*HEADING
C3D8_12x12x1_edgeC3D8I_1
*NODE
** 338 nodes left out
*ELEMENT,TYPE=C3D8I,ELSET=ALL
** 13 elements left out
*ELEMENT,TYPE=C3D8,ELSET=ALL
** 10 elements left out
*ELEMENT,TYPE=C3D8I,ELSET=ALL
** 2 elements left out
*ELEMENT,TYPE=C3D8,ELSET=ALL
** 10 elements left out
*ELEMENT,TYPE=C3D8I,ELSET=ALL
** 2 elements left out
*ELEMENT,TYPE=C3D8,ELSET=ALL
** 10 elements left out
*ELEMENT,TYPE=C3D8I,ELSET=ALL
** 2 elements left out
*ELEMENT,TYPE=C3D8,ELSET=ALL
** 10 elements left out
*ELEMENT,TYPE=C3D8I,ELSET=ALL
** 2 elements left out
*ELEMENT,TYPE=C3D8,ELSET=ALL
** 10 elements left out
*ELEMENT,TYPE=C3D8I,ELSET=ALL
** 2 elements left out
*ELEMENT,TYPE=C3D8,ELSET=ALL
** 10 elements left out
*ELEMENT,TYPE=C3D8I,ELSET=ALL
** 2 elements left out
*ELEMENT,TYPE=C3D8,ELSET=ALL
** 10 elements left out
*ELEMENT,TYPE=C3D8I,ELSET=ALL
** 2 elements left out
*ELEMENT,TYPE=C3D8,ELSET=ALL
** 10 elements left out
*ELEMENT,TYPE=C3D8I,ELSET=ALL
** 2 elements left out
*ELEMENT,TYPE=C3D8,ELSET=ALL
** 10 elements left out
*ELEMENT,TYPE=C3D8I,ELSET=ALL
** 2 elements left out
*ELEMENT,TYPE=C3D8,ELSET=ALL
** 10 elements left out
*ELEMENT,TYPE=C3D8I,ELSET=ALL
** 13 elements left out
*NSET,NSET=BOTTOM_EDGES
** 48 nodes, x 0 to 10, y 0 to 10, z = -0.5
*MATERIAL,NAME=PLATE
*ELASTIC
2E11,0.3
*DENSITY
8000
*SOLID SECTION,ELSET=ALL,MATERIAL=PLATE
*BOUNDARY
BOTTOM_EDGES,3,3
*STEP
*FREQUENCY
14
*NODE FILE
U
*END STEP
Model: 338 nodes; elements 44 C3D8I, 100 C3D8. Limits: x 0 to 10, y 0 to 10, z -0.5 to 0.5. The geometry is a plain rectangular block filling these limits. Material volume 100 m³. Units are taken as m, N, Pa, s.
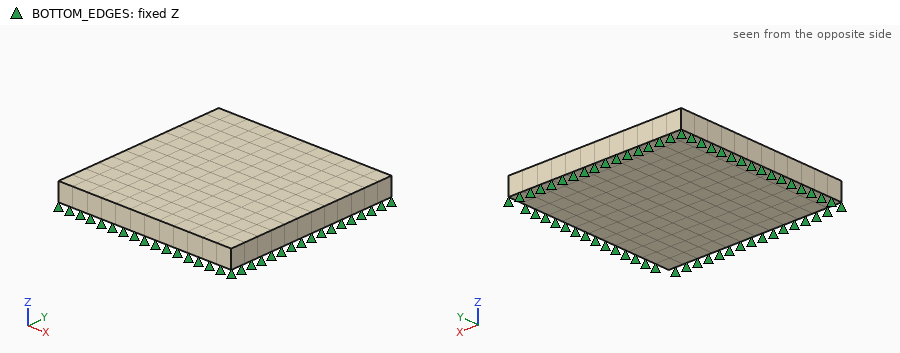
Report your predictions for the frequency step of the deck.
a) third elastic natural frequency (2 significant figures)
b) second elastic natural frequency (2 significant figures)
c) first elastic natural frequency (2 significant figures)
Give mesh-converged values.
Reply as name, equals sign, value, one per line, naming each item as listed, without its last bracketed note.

third elastic natural frequency = 100 Hz
second elastic natural frequency = 100 Hz
first elastic natural frequency = 43 Hz
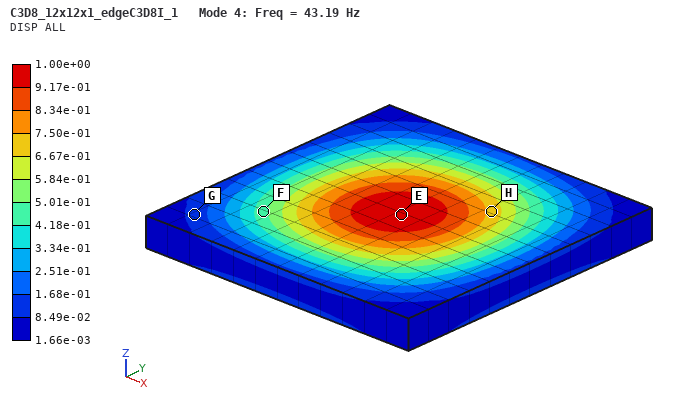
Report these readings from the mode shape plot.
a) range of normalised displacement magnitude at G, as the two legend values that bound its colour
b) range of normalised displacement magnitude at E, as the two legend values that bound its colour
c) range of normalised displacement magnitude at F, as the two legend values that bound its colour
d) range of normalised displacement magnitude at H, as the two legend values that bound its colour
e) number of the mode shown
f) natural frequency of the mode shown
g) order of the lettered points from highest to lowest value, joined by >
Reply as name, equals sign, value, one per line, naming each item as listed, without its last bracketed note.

range of normalised displacement magnitude at G, as the two legend values that bound its colour = 8.49e-02 to 1.68e-01
range of normalised displacement magnitude at E, as the two legend values that bound its colour = 9.17e-01 to 1.00e+00
range of normalised displacement magnitude at F, as the two legend values that bound its colour = 4.18e-01 to 5.01e-01
range of normalised displacement magnitude at H, as the two legend values that bound its colour = 6.67e-01 to 7.50e-01
number of the mode shown = 4
natural frequency of the mode shown = 43.19 Hz
order of the lettered points from highest to lowest value, joined by > = E > H > F > G
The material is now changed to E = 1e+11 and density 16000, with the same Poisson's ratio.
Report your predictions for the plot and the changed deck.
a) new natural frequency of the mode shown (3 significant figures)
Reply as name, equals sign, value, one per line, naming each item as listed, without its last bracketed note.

new natural frequency of the mode shown = 21.6 Hz
